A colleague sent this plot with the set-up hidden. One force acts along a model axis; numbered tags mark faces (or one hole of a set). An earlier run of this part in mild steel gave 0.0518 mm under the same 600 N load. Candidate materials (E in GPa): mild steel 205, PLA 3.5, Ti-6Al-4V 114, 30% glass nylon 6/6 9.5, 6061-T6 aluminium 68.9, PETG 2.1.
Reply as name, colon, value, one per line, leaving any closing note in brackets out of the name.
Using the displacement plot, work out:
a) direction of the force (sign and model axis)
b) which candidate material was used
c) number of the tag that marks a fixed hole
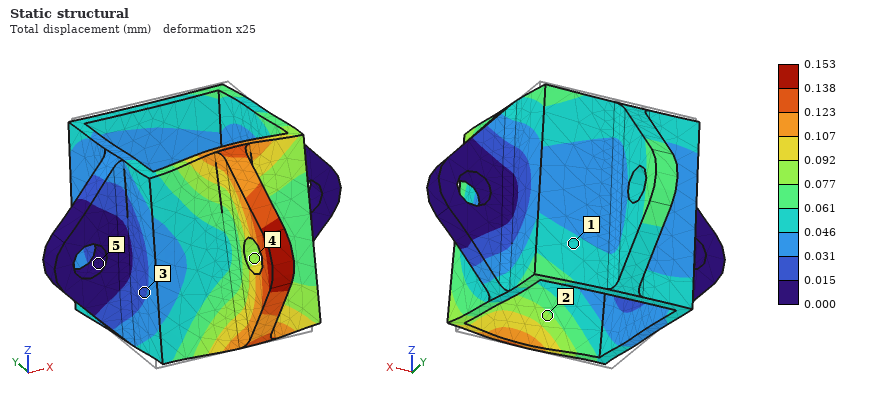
direction of the force: +Z
which candidate material was used: 6061-T6 aluminium
number of the tag that marks a fixed hole: 5
